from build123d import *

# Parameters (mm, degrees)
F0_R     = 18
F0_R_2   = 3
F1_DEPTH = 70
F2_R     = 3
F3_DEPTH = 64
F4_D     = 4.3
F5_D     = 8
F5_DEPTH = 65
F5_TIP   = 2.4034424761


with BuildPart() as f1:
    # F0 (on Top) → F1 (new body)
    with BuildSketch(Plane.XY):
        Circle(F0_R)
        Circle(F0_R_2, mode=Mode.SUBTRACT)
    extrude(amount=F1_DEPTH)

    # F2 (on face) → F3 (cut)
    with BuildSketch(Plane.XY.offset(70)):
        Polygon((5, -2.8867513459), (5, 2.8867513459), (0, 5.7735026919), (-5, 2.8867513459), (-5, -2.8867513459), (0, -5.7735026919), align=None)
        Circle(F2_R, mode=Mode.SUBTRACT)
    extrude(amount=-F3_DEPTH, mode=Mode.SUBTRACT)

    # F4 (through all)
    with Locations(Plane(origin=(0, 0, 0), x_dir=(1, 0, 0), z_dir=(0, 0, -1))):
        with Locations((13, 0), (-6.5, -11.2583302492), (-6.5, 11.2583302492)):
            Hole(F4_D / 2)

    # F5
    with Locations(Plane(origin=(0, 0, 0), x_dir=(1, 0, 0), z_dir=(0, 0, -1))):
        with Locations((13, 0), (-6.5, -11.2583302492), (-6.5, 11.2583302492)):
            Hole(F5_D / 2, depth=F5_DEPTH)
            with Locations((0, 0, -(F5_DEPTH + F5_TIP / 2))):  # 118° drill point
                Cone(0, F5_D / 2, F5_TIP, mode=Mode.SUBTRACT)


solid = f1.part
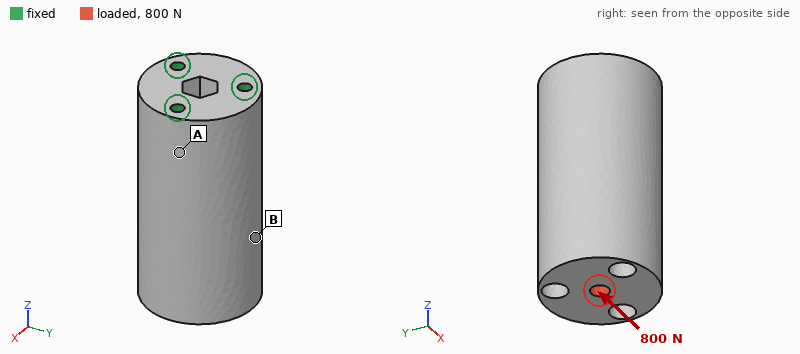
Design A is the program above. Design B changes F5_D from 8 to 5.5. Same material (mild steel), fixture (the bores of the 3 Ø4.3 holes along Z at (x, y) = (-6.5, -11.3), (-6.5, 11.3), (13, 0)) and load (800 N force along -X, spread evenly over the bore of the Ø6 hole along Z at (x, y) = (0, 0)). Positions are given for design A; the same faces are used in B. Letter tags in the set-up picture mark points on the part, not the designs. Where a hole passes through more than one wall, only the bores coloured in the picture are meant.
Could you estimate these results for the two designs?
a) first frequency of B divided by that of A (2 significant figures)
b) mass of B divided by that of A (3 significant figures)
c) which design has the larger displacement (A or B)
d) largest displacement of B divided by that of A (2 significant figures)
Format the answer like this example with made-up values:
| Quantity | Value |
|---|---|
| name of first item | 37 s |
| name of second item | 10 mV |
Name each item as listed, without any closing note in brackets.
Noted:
| Quantity | Value |
|---|---|
| first frequency of B divided by that of A | 1.1 |
| mass of B divided by that of A | 1.09 |
| which design has the larger displacement | A |
| largest displacement of B divided by that of A | 0.75 |
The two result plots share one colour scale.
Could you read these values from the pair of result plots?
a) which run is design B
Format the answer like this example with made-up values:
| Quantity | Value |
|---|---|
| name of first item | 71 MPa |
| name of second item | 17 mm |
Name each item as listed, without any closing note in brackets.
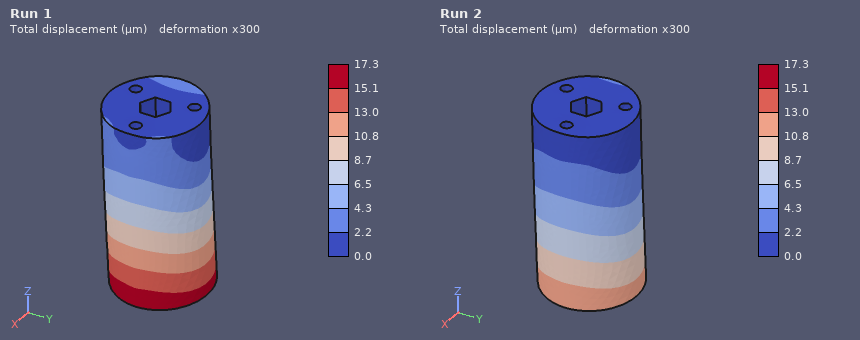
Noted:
| Quantity | Value |
|---|---|
| which run is design B | Run 2 |
